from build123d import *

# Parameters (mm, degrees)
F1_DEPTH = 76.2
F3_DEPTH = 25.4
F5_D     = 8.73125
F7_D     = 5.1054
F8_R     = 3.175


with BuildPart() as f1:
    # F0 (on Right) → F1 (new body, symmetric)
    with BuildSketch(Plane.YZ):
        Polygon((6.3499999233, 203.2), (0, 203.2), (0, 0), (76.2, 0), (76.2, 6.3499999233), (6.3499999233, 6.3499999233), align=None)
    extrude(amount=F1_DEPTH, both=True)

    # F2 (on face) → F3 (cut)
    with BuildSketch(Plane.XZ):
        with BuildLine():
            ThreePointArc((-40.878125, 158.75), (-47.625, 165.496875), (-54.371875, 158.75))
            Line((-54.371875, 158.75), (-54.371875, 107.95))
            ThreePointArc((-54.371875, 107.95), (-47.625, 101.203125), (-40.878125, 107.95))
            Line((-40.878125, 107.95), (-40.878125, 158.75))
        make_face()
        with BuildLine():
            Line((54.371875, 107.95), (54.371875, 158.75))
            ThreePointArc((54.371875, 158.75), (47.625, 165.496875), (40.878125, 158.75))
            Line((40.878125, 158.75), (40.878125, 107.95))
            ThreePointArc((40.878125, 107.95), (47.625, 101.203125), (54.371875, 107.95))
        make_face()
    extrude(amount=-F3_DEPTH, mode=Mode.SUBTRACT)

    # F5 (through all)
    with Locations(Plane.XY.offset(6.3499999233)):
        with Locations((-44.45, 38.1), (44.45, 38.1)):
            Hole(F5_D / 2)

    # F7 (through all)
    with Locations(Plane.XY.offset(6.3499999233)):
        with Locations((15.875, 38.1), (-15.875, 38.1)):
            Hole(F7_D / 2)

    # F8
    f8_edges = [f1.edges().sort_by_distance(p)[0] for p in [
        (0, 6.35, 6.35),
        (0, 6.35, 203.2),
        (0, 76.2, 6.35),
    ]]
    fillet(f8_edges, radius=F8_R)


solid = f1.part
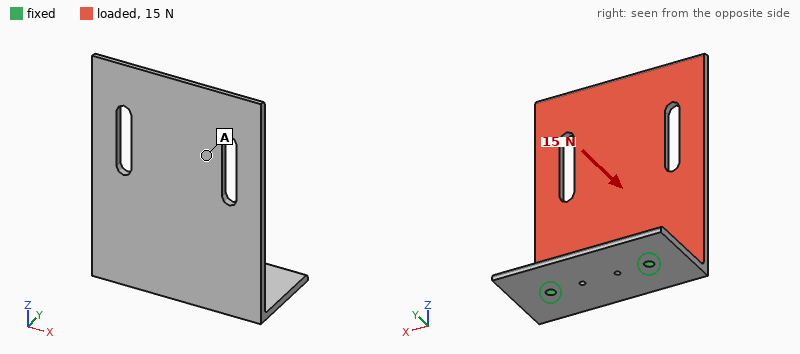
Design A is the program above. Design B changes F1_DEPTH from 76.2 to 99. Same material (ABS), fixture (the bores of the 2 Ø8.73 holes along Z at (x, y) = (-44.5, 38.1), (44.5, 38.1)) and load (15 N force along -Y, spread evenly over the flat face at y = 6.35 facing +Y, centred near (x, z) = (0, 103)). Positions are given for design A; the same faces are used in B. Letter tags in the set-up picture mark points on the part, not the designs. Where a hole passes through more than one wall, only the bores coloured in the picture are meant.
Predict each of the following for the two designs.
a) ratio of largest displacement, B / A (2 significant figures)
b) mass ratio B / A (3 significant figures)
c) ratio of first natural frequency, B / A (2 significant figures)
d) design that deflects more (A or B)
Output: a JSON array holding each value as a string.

["0.81", "1.31", "0.97", "A"]
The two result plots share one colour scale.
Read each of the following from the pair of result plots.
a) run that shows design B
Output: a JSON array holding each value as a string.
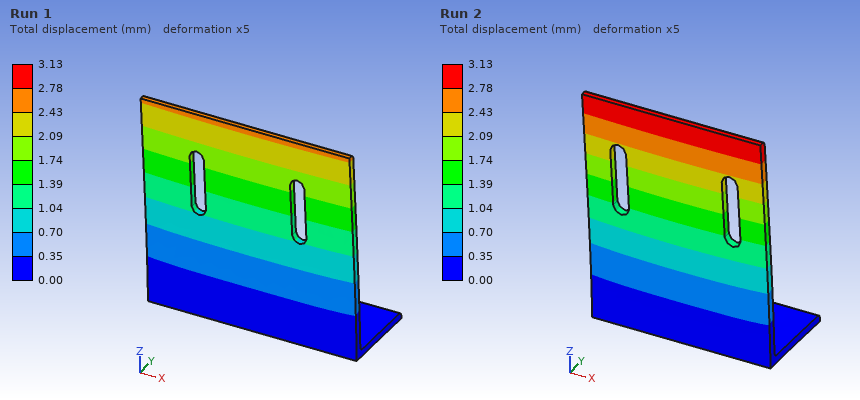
["Run 1"]
